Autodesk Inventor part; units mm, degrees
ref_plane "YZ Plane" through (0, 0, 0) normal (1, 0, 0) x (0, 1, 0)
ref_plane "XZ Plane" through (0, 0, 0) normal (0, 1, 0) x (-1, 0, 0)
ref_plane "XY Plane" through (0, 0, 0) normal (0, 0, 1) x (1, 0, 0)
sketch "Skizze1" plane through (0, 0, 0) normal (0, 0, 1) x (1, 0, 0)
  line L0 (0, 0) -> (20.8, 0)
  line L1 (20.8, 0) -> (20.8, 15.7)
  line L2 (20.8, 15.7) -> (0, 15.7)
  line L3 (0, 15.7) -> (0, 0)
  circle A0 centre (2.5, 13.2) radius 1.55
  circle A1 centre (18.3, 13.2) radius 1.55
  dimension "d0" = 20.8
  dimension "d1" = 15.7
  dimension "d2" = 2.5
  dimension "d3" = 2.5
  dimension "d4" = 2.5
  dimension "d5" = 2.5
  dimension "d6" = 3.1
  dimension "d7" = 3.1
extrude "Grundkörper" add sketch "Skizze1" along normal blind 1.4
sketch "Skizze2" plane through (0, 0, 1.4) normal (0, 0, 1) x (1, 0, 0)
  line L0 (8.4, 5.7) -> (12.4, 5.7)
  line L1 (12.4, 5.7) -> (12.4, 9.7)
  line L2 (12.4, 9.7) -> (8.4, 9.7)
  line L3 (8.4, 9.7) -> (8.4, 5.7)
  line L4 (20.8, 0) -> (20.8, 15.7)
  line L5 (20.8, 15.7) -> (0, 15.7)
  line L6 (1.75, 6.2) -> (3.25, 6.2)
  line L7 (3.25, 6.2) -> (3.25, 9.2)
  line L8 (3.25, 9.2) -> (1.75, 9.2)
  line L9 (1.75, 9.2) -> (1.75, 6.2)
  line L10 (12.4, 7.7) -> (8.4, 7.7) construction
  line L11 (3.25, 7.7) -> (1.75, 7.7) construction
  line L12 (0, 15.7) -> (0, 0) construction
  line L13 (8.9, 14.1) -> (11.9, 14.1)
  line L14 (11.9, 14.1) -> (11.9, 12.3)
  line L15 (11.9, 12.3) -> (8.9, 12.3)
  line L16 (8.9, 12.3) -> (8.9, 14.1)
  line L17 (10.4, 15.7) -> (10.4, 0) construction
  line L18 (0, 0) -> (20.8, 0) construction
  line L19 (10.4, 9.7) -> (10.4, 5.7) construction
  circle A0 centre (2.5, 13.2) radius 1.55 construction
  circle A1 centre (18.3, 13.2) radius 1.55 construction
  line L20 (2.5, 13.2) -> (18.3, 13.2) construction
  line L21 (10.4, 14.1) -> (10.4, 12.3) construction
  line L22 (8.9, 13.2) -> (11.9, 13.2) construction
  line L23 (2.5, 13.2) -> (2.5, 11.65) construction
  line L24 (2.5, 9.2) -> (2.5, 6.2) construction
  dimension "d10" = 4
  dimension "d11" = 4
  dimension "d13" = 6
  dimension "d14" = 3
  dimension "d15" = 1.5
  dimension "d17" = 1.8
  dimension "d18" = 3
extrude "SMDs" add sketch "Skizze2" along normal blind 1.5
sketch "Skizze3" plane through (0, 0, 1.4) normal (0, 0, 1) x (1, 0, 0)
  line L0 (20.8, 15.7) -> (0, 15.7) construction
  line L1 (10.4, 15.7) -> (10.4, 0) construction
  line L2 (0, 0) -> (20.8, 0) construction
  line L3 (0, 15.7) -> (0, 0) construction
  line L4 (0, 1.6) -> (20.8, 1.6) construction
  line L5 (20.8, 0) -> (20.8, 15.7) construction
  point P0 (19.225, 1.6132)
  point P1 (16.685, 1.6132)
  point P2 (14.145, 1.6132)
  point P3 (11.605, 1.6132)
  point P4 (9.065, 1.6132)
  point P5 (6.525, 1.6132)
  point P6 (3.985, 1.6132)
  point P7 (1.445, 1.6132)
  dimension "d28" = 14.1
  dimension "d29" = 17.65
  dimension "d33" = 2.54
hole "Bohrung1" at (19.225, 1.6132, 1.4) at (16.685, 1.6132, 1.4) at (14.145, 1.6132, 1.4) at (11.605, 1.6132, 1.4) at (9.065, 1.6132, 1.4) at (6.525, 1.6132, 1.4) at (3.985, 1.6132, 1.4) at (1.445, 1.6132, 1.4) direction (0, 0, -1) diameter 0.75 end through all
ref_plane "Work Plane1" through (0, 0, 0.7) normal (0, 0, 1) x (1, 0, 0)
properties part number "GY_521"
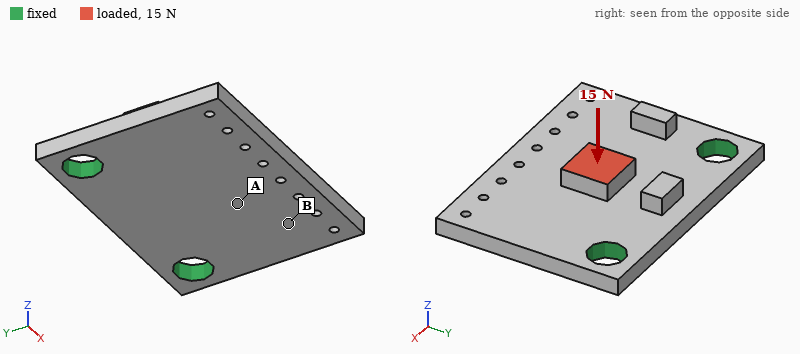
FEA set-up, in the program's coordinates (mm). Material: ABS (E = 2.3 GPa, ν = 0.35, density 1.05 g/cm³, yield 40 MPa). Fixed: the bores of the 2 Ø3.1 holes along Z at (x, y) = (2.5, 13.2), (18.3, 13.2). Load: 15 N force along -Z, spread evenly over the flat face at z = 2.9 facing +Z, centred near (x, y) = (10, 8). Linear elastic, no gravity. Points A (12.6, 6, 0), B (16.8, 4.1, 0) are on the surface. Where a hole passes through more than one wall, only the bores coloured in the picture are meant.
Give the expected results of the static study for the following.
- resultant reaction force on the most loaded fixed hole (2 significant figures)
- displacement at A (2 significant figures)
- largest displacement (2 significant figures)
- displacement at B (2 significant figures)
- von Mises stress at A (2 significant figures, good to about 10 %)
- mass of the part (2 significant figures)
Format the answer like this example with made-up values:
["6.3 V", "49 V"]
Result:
["7.6 N", "0.14 mm", "0.27 mm", "0.14 mm", "4.9 MPa", "0.49 g"]
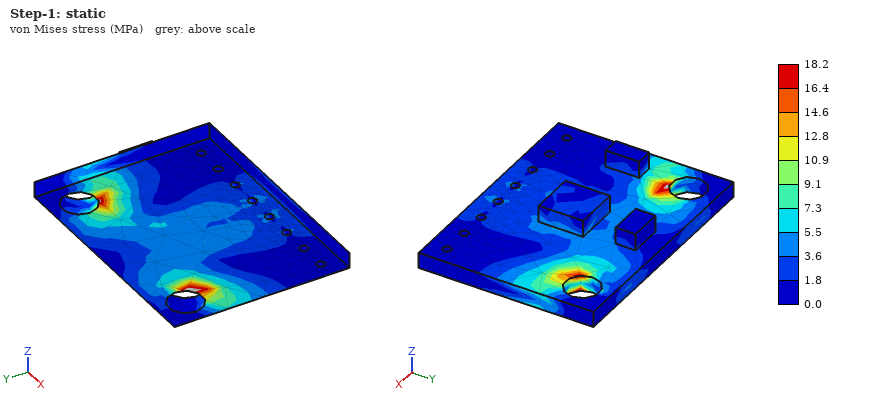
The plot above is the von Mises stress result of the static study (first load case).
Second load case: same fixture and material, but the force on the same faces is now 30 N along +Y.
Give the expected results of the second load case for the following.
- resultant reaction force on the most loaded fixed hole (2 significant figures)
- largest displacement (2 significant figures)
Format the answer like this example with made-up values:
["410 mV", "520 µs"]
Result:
["16 N", "0.31 mm"]
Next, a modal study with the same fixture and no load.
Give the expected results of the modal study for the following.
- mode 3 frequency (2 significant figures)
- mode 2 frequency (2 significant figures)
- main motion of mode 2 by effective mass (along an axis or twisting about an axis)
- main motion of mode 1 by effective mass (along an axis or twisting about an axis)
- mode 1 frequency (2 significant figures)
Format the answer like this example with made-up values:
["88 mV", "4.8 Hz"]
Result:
["7300 Hz", "4000 Hz", "twisting about Y", "along Z", "2100 Hz"]
